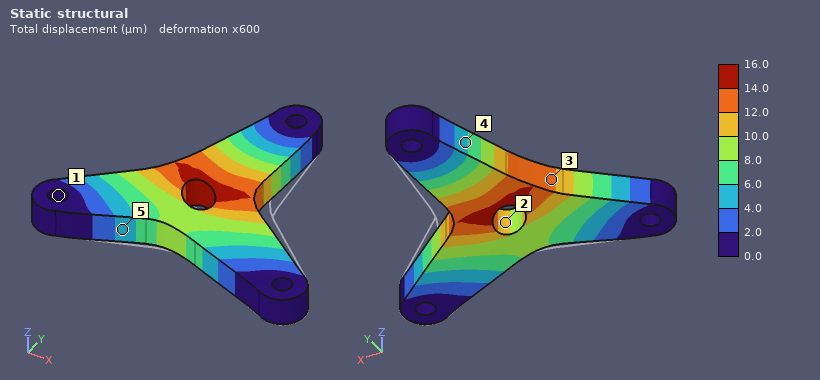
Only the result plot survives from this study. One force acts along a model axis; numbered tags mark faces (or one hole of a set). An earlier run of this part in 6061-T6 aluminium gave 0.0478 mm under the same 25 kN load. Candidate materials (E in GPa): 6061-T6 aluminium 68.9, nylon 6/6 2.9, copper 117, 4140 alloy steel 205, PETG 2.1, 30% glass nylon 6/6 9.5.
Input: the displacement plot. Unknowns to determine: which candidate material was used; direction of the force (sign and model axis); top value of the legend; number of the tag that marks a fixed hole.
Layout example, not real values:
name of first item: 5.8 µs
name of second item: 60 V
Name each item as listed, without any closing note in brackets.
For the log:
which candidate material was used: 4140 alloy steel
direction of the force: -X
top value of the legend: 16.0 µm
number of the tag that marks a fixed hole: 1
